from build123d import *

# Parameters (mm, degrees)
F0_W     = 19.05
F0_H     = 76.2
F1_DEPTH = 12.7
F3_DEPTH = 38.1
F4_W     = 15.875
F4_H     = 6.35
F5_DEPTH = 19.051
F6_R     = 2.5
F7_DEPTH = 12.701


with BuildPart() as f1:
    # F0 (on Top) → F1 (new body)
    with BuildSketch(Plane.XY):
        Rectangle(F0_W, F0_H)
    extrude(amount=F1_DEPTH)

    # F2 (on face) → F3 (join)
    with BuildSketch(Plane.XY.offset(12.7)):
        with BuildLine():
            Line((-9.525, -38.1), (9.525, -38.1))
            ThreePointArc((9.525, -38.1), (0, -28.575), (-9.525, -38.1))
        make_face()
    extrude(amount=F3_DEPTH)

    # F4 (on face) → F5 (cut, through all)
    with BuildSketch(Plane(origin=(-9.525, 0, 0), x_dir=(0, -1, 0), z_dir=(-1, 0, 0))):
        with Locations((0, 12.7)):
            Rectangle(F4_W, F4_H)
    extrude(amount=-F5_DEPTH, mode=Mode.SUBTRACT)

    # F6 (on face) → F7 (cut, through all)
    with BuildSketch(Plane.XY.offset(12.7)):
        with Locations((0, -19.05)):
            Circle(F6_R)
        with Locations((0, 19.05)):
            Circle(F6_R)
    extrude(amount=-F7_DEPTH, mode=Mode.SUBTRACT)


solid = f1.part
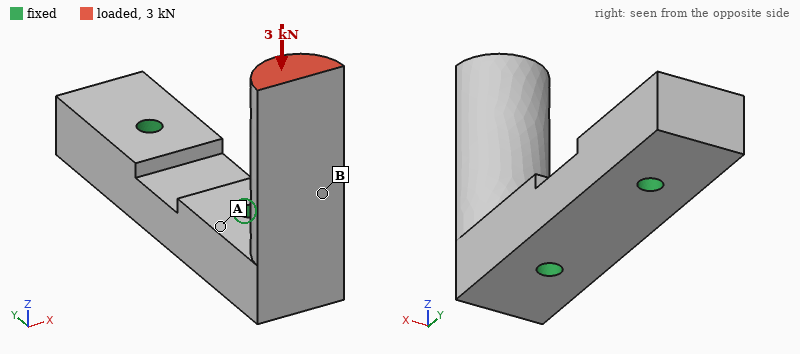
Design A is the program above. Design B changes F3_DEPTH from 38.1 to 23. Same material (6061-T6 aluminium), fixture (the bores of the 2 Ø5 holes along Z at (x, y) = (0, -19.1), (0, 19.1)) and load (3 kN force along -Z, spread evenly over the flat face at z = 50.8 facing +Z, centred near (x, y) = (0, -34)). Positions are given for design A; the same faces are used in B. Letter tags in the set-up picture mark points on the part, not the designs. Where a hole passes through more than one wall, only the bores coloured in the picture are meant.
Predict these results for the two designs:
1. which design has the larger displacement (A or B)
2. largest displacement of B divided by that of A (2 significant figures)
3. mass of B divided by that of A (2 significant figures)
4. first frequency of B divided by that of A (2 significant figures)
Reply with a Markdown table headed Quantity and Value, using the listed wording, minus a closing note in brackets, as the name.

| Quantity | Value |
|---|---|
| which design has the larger displacement | A |
| largest displacement of B divided by that of A | 0.71 |
| mass of B divided by that of A | 0.90 |
| first frequency of B divided by that of A | 2.1 |
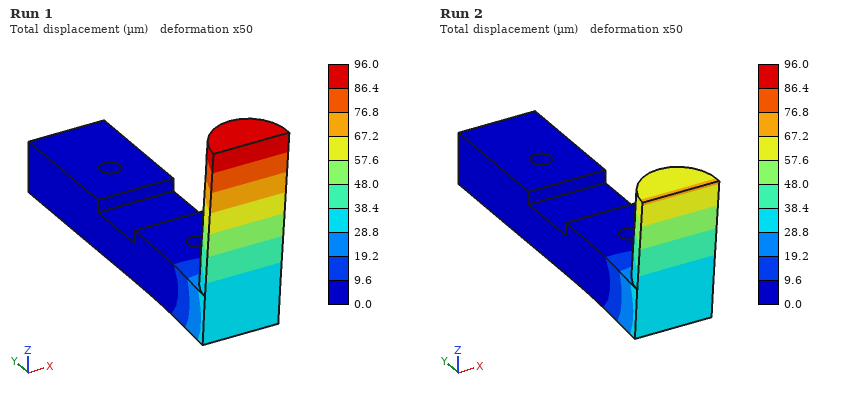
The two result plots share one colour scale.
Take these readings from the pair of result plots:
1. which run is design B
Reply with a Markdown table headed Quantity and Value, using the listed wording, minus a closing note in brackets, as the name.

| Quantity | Value |
|---|---|
| which run is design B | Run 2 |
